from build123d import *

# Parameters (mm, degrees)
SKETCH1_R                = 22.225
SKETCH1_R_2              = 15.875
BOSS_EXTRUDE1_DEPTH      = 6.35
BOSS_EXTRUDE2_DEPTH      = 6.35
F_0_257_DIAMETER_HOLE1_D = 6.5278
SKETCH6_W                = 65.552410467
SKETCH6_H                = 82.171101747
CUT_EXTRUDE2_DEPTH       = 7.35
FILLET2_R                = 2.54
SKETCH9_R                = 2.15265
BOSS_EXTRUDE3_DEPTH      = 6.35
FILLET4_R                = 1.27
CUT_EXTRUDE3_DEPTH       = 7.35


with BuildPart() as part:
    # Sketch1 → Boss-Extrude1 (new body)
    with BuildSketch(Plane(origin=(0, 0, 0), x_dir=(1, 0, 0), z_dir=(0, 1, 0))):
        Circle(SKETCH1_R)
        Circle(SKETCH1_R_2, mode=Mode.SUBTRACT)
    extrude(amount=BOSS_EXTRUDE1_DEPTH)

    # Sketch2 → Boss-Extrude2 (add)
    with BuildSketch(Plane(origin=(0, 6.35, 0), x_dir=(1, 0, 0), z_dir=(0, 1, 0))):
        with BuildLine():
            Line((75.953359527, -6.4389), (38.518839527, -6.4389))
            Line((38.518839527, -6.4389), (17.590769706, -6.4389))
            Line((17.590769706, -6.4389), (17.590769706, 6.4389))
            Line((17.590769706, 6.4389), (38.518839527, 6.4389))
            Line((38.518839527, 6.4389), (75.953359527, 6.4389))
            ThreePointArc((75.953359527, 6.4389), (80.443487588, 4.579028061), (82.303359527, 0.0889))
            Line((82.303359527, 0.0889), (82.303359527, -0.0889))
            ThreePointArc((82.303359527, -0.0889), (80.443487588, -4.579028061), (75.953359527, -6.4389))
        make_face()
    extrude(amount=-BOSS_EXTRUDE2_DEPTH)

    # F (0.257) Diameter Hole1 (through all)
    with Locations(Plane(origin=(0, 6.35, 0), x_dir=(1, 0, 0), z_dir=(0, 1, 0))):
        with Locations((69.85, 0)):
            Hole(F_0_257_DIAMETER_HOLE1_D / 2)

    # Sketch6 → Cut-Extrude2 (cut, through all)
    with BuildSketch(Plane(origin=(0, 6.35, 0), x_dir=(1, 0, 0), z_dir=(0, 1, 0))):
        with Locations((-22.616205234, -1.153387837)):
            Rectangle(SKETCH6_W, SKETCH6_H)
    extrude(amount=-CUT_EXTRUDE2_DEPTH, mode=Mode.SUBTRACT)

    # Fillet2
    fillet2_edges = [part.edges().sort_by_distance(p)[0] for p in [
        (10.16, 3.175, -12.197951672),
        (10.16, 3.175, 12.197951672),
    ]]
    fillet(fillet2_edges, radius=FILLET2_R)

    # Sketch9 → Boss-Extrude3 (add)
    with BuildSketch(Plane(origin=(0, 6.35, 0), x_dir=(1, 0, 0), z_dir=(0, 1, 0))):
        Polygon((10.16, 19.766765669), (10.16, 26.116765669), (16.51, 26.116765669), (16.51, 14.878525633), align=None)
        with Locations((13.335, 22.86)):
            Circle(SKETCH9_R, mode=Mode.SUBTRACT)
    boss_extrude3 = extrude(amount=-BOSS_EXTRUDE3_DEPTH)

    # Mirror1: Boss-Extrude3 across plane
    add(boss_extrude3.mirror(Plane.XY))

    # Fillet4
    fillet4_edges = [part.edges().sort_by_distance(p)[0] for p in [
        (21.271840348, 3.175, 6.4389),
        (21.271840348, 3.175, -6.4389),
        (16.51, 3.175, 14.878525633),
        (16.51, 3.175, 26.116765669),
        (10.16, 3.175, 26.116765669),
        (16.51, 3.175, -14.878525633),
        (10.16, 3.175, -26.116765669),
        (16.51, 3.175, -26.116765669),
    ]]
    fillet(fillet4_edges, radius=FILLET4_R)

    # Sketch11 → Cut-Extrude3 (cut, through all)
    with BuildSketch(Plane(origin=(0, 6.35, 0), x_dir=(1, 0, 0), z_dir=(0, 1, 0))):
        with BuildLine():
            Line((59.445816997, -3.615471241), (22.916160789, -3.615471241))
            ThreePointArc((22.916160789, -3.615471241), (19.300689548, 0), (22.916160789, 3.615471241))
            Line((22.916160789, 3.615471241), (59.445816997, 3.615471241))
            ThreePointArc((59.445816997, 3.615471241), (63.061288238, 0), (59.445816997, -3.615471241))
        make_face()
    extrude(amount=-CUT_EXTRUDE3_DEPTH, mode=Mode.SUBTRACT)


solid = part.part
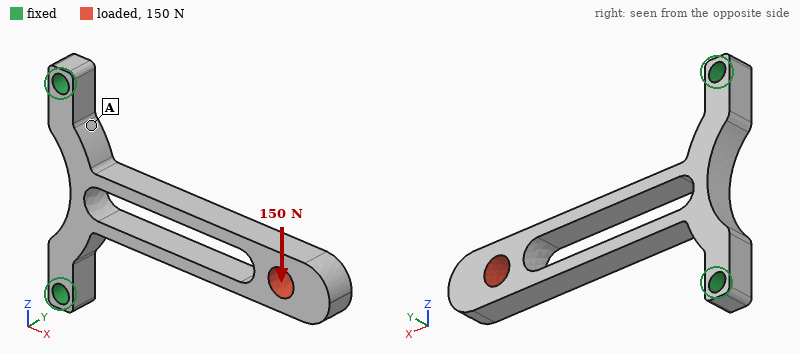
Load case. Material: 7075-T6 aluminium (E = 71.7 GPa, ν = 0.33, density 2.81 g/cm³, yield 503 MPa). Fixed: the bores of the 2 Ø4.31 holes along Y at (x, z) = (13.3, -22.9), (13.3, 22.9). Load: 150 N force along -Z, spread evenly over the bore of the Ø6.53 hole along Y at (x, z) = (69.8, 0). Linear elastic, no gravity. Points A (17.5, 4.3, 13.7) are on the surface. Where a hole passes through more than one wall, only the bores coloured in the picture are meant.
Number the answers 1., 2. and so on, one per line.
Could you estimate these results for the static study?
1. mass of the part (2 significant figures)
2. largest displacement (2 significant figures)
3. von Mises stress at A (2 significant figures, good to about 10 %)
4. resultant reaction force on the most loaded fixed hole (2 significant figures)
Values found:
1. 13 g
2. 0.71 mm
3. 27 MPa
4. 280 N
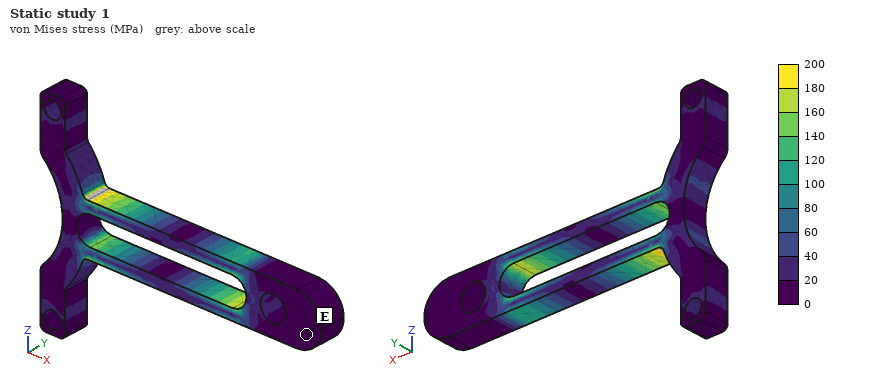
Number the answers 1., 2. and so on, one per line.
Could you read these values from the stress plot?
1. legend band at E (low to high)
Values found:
1. 0 to 20 MPa
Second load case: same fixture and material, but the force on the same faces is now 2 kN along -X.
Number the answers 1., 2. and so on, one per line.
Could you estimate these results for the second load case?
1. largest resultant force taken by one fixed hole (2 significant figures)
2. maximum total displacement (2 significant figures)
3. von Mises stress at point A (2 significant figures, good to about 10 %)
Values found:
1. 2.0 kN
2. 94 µm
3. 52 MPa
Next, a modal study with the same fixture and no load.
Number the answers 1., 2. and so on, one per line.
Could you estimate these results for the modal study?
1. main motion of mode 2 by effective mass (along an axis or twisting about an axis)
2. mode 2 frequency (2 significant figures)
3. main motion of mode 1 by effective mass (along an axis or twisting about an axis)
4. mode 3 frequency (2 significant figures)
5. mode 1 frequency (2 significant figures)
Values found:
1. along Z
2. 1100 Hz
3. along Y
4. 3800 Hz
5. 760 Hz
